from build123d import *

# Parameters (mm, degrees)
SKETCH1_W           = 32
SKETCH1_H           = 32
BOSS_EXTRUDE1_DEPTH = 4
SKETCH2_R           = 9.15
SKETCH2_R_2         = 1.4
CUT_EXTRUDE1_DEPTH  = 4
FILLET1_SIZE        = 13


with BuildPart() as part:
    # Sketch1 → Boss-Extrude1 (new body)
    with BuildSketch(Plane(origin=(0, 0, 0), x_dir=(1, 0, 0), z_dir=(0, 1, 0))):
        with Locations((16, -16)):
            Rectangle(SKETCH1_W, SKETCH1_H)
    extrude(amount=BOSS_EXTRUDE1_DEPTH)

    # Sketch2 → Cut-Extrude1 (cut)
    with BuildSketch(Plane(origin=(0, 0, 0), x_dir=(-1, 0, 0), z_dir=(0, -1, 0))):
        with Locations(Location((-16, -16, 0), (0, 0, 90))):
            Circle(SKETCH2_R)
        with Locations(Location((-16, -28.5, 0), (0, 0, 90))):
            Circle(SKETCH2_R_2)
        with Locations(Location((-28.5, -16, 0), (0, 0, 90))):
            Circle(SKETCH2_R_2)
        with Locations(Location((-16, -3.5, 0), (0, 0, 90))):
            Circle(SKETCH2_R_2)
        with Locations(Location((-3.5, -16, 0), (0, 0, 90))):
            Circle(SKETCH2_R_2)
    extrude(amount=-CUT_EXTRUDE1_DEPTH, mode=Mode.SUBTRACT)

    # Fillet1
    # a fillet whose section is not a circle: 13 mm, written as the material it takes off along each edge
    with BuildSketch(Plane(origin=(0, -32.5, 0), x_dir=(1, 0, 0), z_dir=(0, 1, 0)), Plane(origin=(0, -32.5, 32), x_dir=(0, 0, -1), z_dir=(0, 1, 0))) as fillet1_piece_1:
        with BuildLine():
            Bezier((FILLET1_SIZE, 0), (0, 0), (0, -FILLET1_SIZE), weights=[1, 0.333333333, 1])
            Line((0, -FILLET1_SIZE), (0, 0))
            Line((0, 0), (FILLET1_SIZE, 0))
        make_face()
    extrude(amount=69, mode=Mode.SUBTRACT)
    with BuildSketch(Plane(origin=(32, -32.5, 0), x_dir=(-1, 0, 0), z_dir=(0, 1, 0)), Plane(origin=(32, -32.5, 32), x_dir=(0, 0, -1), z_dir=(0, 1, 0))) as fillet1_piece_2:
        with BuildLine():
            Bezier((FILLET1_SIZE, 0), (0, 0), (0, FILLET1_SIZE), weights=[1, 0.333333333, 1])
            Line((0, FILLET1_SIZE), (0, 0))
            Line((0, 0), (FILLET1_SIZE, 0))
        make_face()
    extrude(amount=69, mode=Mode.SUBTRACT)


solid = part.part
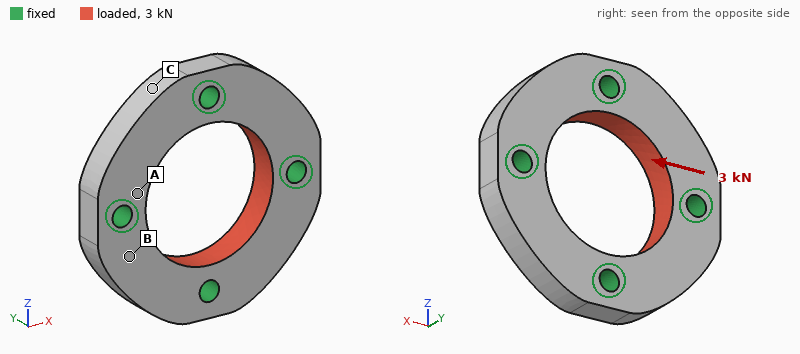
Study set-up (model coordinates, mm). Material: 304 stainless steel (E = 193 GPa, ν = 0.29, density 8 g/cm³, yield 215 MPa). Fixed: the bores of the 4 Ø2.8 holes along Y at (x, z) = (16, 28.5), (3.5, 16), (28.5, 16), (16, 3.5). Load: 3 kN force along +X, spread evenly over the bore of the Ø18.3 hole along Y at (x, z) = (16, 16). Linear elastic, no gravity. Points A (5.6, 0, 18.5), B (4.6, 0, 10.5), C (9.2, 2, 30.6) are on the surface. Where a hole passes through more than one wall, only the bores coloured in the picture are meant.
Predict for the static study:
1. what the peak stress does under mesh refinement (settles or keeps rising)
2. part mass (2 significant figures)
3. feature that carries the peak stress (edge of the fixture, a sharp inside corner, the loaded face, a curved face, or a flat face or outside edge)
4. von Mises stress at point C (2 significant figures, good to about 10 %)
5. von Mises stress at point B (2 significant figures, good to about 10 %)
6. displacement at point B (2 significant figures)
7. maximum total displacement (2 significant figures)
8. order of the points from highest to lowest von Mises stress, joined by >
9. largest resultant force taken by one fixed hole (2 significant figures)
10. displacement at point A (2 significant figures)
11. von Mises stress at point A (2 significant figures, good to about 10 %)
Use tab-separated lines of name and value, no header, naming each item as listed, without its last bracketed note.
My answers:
what the peak stress does under mesh refinement	keeps rising
part mass	17 g
feature that carries the peak stress	edge of the fixture
von Mises stress at point C	6.9 MPa
von Mises stress at point B	14 MPa
displacement at point B	0.78 µm
maximum total displacement	1.2 µm
order of the points from highest to lowest von Mises stress, joined by >	A > B > C
largest resultant force taken by one fixed hole	860 N
displacement at point A	0.46 µm
von Mises stress at point A	24 MPa
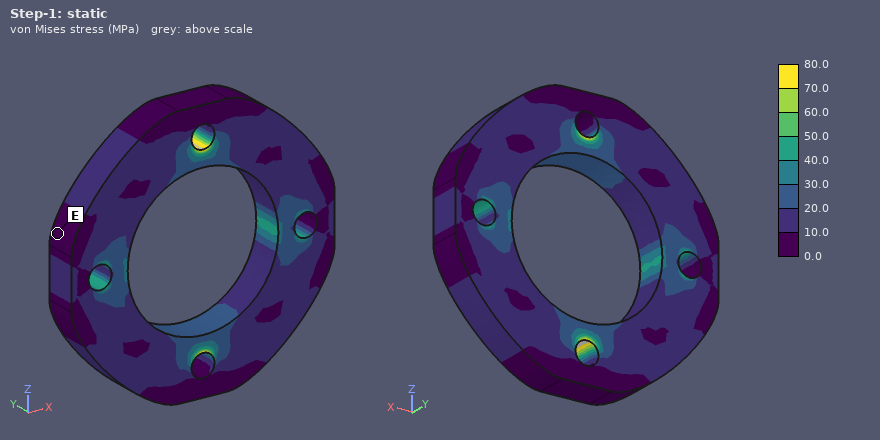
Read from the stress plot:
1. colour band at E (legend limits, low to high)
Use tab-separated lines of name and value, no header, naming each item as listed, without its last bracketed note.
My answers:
colour band at E	0.0 to 10.0 MPa
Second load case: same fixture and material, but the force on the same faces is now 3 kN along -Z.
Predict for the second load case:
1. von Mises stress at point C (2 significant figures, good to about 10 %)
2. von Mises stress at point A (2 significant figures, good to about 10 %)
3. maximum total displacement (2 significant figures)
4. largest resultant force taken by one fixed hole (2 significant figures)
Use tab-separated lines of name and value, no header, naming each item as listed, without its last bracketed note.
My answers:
von Mises stress at point C	8.3 MPa
von Mises stress at point A	24 MPa
maximum total displacement	1.2 µm
largest resultant force taken by one fixed hole	860 N
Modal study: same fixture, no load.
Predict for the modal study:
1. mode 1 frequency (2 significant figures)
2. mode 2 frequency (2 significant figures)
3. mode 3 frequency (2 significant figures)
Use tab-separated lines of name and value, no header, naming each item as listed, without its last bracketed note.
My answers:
mode 1 frequency	41 kHz
mode 2 frequency	42 kHz
mode 3 frequency	42 kHz
